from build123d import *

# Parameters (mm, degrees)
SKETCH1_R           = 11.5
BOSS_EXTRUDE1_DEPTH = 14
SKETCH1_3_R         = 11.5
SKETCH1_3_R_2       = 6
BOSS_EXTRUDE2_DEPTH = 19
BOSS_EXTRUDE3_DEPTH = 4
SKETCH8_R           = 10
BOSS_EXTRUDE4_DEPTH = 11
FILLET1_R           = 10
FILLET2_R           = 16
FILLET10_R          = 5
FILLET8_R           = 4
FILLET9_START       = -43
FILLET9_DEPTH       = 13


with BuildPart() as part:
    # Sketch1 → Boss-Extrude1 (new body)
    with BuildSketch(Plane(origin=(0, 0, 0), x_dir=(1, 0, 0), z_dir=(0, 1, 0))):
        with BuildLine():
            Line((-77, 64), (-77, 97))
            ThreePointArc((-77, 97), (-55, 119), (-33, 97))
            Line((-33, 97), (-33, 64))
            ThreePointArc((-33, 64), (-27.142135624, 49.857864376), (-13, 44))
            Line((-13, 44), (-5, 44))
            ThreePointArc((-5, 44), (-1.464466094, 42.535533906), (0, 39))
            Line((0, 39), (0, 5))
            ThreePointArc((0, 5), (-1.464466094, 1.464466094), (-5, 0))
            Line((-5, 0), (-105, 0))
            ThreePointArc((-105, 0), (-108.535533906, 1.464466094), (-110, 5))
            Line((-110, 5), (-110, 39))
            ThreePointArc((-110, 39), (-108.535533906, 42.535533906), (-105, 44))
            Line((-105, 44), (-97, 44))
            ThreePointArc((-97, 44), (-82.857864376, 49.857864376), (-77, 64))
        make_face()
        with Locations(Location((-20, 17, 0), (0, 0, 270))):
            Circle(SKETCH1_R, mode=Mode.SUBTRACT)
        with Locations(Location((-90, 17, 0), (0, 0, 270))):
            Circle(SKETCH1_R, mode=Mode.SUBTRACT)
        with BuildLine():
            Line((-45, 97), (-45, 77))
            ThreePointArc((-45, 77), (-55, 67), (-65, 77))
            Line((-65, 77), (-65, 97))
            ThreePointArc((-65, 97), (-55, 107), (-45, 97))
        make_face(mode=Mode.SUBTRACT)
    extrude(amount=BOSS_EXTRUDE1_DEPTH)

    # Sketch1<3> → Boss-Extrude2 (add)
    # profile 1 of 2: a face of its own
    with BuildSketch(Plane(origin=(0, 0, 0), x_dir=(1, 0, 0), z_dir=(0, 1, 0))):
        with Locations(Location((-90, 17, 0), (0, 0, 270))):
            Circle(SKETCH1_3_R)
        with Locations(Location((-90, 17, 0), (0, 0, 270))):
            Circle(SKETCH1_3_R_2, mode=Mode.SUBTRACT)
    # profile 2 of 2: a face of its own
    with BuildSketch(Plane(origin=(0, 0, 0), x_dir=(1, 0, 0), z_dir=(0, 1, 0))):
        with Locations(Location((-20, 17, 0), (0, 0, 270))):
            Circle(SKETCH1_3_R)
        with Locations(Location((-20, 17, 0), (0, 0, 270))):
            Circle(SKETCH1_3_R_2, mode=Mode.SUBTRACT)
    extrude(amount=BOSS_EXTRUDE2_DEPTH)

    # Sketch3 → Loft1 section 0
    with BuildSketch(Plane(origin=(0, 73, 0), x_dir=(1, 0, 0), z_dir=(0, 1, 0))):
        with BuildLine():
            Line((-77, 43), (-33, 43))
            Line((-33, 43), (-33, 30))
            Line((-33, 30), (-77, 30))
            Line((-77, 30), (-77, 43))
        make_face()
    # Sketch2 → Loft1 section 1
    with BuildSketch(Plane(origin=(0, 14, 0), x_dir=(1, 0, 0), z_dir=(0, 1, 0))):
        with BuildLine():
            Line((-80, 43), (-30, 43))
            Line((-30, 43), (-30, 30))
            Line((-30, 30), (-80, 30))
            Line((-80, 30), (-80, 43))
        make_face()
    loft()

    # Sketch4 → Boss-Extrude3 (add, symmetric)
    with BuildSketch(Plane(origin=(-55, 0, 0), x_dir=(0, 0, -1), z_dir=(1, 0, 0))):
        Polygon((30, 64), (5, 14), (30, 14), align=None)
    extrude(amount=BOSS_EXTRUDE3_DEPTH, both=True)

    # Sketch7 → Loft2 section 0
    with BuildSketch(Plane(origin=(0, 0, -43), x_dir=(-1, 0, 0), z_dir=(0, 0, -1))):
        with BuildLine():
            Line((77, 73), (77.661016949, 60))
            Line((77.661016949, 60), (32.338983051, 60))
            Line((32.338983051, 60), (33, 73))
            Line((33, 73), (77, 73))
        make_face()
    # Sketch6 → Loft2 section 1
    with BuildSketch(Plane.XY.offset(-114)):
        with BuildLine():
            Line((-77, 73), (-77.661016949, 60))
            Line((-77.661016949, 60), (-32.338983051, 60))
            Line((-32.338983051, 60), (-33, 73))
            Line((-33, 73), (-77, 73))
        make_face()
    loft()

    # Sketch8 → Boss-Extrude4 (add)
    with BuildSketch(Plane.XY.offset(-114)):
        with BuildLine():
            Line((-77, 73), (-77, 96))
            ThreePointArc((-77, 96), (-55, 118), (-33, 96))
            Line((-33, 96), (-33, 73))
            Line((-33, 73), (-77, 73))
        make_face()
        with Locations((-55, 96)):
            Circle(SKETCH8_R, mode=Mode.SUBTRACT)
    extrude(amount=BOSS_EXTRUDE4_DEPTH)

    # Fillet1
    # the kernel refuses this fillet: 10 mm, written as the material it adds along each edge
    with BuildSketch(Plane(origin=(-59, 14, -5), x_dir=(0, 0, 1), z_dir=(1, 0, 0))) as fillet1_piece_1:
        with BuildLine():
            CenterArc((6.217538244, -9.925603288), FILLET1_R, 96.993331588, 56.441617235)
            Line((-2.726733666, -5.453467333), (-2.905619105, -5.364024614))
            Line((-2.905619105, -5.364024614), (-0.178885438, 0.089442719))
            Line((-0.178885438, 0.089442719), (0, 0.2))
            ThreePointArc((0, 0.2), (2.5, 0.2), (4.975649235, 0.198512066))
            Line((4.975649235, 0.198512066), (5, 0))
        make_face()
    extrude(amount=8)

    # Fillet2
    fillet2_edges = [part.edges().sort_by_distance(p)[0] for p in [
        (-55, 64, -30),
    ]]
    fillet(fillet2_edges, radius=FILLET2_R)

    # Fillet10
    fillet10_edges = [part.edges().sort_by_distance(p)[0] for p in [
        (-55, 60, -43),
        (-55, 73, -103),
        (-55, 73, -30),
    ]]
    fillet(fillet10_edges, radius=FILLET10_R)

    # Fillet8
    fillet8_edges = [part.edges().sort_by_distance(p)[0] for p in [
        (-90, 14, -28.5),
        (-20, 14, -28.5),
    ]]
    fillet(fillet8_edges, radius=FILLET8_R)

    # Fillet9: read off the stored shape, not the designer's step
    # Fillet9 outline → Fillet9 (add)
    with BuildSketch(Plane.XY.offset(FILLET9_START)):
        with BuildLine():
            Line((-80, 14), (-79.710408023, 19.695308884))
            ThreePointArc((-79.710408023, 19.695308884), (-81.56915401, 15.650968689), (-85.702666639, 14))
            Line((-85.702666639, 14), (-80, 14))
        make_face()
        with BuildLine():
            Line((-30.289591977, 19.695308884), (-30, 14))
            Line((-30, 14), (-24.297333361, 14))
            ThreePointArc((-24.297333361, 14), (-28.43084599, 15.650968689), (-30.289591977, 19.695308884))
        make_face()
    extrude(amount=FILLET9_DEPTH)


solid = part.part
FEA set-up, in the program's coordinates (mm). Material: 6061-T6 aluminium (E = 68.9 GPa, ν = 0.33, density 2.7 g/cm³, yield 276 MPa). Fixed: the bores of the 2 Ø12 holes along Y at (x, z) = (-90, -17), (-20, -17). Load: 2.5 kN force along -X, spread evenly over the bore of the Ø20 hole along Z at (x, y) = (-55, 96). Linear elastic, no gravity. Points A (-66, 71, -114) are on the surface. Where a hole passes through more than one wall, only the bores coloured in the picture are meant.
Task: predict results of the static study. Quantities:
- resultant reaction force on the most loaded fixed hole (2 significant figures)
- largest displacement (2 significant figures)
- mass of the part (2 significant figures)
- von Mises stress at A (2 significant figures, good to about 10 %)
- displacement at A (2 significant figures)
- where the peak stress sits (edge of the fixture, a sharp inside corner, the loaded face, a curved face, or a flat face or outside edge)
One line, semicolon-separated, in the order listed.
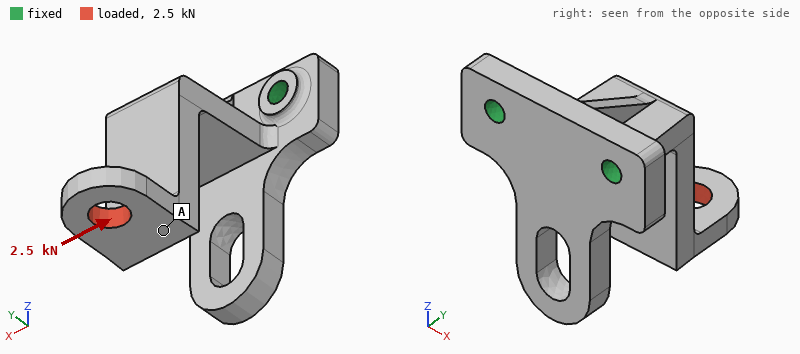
5.0 kN; 0.99 mm; 550 g; 19 MPa; 0.72 mm; a sharp inside corner
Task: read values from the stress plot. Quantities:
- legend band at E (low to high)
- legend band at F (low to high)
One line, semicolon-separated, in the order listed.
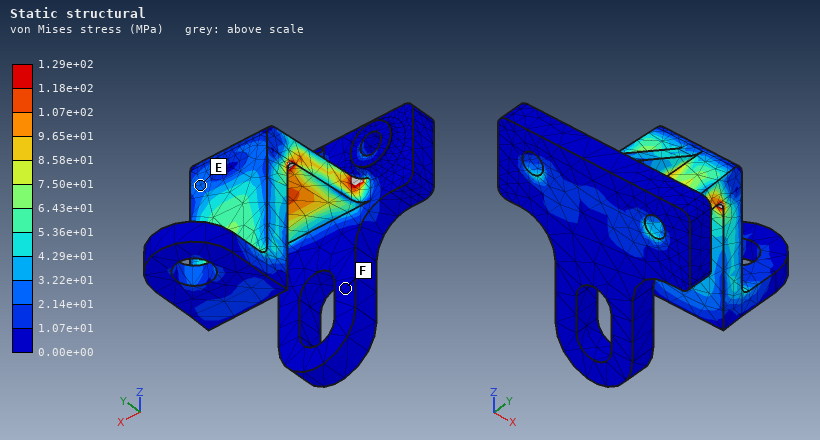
2.14e+01 to 3.22e+01 MPa; 0.00e+00 to 1.07e+01 MPa
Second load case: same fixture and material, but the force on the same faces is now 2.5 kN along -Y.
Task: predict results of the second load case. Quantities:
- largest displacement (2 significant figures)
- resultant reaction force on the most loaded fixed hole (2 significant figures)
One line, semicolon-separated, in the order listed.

1.8 mm; 1.4 kN
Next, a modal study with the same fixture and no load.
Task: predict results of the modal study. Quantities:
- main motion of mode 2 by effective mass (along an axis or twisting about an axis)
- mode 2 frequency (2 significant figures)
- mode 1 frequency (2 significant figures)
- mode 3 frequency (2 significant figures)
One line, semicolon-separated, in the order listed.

along X; 970 Hz; 670 Hz; 1700 Hz
